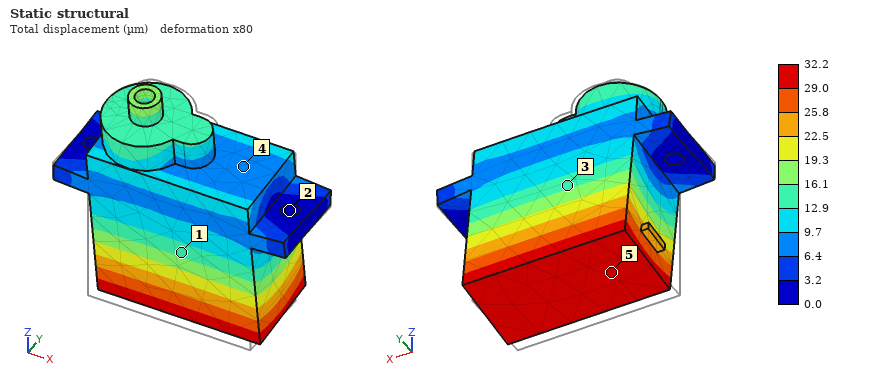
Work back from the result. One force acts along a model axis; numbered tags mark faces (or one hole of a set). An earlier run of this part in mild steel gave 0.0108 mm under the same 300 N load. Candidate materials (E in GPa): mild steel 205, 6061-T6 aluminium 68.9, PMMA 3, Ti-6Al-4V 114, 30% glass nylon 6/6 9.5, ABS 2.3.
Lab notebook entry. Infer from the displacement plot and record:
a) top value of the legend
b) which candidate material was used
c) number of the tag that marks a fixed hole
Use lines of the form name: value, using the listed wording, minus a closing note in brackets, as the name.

top value of the legend: 32.2 µm
which candidate material was used: 6061-T6 aluminium
number of the tag that marks a fixed hole: 2
